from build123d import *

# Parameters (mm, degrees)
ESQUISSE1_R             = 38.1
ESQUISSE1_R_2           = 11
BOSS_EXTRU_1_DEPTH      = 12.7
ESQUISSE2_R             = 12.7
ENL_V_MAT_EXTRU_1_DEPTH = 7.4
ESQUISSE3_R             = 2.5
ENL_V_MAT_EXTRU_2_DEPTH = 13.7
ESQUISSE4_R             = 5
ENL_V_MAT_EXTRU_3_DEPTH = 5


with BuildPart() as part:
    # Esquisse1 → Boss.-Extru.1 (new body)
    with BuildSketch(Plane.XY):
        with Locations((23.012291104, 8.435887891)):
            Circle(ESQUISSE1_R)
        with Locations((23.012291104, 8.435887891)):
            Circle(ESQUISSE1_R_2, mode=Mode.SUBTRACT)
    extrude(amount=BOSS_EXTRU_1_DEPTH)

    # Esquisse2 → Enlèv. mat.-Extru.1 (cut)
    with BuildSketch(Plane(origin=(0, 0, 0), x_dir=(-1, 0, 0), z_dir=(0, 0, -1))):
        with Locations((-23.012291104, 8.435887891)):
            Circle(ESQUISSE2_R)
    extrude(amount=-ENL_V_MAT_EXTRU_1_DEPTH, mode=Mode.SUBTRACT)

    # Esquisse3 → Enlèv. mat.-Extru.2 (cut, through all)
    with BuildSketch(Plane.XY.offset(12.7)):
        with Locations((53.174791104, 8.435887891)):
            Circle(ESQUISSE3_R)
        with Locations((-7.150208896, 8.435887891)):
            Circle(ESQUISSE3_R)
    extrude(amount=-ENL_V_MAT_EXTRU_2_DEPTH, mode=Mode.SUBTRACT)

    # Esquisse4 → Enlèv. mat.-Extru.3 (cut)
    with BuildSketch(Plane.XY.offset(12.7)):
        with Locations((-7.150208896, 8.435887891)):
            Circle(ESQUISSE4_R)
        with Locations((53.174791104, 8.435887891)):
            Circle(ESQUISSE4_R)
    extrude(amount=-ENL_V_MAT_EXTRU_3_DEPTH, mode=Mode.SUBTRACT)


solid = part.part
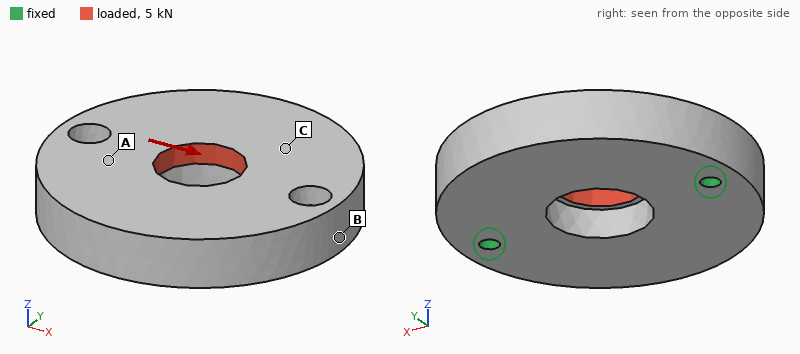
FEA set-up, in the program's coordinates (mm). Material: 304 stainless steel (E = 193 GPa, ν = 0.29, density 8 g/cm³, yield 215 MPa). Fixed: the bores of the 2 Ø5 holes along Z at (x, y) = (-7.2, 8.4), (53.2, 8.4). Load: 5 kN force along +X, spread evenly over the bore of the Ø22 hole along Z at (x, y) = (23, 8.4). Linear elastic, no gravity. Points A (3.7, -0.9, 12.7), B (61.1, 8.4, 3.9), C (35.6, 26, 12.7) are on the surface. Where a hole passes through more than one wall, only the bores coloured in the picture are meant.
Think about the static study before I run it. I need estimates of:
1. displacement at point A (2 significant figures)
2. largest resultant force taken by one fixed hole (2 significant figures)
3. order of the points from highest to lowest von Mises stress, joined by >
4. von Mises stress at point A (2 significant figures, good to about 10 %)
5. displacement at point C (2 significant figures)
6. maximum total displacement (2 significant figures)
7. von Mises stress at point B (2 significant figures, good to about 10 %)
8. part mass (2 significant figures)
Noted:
1.4 µm
2.5 kN
B > A > C
7.9 MPa
1.5 µm
2.2 µm
14 MPa
410 g
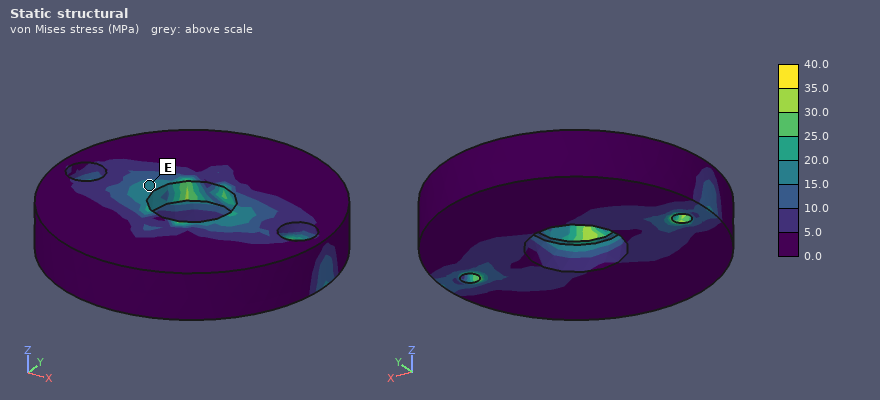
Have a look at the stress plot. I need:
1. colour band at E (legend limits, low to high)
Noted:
15.0 to 20.0 MPa
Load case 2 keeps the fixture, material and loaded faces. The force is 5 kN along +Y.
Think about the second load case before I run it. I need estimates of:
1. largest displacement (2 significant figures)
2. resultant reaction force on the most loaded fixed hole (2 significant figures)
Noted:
16 µm
2.5 kN
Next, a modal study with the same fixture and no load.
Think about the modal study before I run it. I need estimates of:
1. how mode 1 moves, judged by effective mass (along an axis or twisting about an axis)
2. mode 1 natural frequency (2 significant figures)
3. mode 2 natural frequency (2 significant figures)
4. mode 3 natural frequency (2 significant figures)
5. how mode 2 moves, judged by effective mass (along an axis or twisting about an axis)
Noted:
twisting about X
3400 Hz
5600 Hz
11 kHz
along Z
